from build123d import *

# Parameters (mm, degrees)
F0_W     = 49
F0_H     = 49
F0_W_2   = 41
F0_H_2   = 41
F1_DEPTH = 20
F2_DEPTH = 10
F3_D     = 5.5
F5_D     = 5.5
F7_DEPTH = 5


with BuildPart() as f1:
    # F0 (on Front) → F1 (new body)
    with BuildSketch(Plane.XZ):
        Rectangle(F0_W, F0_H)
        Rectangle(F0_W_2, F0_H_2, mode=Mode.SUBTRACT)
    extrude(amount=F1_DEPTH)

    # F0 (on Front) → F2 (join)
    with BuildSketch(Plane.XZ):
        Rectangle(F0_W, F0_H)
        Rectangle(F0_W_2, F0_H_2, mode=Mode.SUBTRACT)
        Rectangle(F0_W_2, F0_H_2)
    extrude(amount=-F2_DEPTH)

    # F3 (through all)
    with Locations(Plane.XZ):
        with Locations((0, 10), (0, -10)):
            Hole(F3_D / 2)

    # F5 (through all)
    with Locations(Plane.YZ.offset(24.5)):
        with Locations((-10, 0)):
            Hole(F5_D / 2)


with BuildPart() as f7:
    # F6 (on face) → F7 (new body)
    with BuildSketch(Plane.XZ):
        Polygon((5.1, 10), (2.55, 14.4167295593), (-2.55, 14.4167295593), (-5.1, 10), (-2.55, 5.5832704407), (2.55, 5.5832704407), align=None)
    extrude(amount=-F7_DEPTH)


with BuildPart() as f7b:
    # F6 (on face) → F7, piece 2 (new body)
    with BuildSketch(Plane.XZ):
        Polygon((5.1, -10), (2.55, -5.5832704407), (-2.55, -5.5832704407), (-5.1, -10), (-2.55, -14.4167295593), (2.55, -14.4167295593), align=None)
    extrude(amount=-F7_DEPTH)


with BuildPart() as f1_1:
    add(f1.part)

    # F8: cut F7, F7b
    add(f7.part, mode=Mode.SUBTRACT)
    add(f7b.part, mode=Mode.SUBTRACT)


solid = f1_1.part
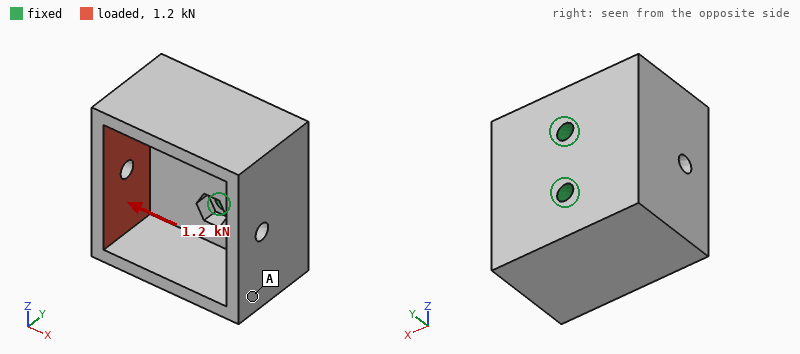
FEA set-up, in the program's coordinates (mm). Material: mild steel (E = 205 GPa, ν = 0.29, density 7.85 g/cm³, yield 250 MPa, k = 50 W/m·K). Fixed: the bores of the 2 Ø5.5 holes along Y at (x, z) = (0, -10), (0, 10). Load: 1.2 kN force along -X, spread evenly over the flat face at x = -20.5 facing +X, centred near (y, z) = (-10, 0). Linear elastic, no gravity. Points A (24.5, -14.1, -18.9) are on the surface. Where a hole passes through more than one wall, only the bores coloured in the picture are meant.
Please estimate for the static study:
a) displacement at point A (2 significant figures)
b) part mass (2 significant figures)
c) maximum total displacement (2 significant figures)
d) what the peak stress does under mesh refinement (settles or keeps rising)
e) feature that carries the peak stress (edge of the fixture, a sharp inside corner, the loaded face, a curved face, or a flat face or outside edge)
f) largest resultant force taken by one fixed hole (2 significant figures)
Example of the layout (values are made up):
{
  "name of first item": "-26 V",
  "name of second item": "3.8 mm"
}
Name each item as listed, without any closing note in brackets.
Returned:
{
  "displacement at point A": "14 µm",
  "part mass": "290 g",
  "maximum total displacement": "31 µm",
  "what the peak stress does under mesh refinement": "keeps rising",
  "feature that carries the peak stress": "edge of the fixture",
  "largest resultant force taken by one fixed hole": "610 N"
}
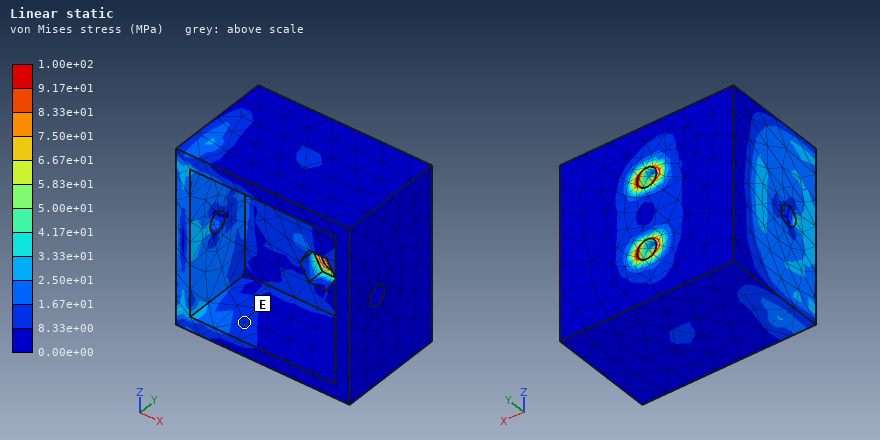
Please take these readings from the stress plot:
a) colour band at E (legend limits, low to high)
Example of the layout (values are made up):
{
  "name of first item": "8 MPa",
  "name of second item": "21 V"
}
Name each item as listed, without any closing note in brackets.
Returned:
{
  "colour band at E": "8.33e+00 to 1.67e+01 MPa"
}
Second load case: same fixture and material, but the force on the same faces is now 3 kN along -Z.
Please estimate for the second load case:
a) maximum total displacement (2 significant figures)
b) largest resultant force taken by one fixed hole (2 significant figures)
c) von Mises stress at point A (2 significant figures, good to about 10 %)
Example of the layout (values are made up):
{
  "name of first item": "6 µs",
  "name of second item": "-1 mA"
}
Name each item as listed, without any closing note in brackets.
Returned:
{
  "maximum total displacement": "28 µm",
  "largest resultant force taken by one fixed hole": "3.7 kN",
  "von Mises stress at point A": "13 MPa"
}
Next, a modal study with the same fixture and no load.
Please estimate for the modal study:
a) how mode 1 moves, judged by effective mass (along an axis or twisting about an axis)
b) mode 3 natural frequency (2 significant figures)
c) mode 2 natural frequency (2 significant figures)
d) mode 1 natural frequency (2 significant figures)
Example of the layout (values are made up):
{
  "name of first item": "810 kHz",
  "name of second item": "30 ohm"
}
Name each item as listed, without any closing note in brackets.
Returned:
{
  "how mode 1 moves, judged by effective mass": "along X",
  "mode 3 natural frequency": "6600 Hz",
  "mode 2 natural frequency": "6400 Hz",
  "mode 1 natural frequency": "3200 Hz"
}
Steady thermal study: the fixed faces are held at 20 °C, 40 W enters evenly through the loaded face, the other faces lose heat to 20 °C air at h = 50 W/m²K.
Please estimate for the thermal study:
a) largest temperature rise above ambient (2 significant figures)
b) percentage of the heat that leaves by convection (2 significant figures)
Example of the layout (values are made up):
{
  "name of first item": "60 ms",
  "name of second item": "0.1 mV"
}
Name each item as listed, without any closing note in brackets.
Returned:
{
  "largest temperature rise above ambient": "69 K",
  "percentage of the heat that leaves by convection": "29 %"
}
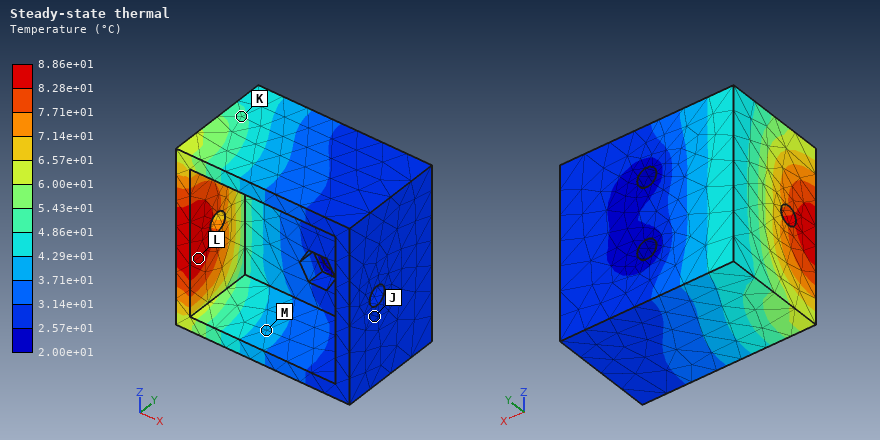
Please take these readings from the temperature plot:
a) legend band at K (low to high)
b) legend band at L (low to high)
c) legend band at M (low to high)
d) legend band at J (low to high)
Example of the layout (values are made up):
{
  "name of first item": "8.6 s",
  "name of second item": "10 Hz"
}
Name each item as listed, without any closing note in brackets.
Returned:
{
  "legend band at K": "4.86e+01 to 5.43e+01 °C",
  "legend band at L": "8.28e+01 to 8.86e+01 °C",
  "legend band at M": "3.71e+01 to 4.29e+01 °C",
  "legend band at J": "2.57e+01 to 3.14e+01 °C"
}
